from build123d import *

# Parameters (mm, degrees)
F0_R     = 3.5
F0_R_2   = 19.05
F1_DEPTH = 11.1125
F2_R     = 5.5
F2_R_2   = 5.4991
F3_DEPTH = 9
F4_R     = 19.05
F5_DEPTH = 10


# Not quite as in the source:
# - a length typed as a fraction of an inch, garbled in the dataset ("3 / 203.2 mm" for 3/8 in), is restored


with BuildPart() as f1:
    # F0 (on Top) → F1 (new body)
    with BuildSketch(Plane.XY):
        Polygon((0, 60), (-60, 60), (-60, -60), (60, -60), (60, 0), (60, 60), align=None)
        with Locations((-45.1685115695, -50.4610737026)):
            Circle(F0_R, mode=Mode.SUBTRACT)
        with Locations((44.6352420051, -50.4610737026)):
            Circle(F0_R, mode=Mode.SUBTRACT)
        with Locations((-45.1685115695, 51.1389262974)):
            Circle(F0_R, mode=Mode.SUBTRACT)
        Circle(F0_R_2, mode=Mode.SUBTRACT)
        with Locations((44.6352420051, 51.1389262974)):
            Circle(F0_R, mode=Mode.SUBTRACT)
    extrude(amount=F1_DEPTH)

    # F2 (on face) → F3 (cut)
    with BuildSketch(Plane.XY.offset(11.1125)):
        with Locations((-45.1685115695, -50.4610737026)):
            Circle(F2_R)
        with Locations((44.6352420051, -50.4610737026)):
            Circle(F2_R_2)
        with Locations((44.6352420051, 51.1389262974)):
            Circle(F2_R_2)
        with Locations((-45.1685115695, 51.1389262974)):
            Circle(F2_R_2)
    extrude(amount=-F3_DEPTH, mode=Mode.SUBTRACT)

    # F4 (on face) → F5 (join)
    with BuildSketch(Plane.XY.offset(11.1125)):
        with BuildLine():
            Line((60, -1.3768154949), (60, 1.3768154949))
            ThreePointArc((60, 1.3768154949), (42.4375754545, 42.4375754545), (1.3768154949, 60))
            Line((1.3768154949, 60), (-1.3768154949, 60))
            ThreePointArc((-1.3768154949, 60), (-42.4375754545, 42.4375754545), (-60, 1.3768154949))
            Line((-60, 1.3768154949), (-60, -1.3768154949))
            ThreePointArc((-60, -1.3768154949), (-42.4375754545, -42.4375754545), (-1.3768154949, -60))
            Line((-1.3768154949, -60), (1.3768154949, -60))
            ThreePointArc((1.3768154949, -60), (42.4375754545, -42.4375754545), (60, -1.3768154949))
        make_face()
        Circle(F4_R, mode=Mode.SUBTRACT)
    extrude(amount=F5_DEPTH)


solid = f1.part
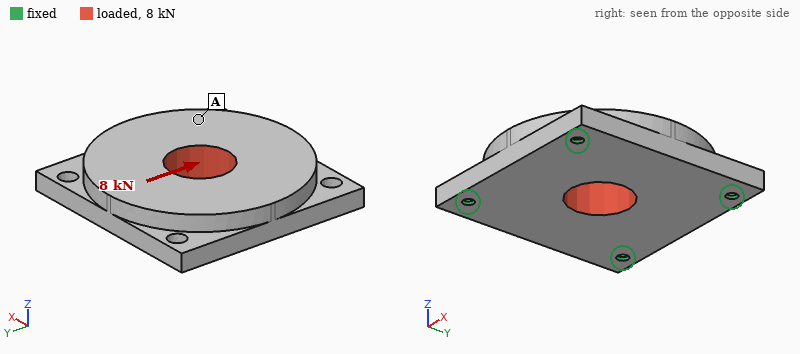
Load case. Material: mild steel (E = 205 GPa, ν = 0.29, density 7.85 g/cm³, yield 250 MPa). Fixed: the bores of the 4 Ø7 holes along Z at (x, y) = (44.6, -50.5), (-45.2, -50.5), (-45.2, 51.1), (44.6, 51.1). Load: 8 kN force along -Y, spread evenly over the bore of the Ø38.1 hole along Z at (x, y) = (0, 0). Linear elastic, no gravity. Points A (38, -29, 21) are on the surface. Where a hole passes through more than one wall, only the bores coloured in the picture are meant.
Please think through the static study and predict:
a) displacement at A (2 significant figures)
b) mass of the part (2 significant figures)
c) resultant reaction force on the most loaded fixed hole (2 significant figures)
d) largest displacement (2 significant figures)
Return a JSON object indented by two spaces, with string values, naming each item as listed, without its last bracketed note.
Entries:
{
  "displacement at A": "2.2 µm",
  "mass of the part": "1.9 kg",
  "resultant reaction force on the most loaded fixed hole": "2.1 kN",
  "largest displacement": "3.1 µm"
}
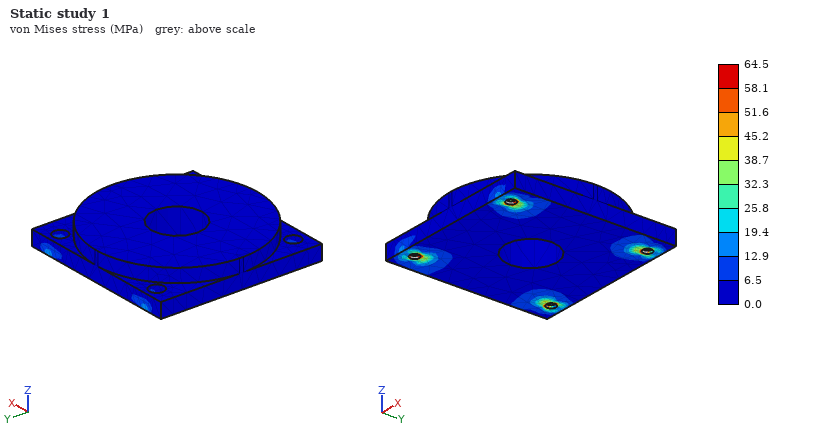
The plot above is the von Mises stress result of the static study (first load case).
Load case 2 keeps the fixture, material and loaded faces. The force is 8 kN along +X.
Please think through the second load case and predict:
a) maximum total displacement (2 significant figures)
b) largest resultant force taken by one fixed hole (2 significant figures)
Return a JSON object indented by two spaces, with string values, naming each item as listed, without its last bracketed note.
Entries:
{
  "maximum total displacement": "3.3 µm",
  "largest resultant force taken by one fixed hole": "2.1 kN"
}
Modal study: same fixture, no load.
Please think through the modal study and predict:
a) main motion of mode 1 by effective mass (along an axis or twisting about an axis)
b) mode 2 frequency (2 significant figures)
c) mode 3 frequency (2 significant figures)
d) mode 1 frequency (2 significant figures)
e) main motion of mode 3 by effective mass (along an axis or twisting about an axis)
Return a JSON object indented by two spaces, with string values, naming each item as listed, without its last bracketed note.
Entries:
{
  "main motion of mode 1 by effective mass": "along Z",
  "mode 2 frequency": "5300 Hz",
  "mode 3 frequency": "6300 Hz",
  "mode 1 frequency": "3900 Hz",
  "main motion of mode 3 by effective mass": "twisting about X"
}
